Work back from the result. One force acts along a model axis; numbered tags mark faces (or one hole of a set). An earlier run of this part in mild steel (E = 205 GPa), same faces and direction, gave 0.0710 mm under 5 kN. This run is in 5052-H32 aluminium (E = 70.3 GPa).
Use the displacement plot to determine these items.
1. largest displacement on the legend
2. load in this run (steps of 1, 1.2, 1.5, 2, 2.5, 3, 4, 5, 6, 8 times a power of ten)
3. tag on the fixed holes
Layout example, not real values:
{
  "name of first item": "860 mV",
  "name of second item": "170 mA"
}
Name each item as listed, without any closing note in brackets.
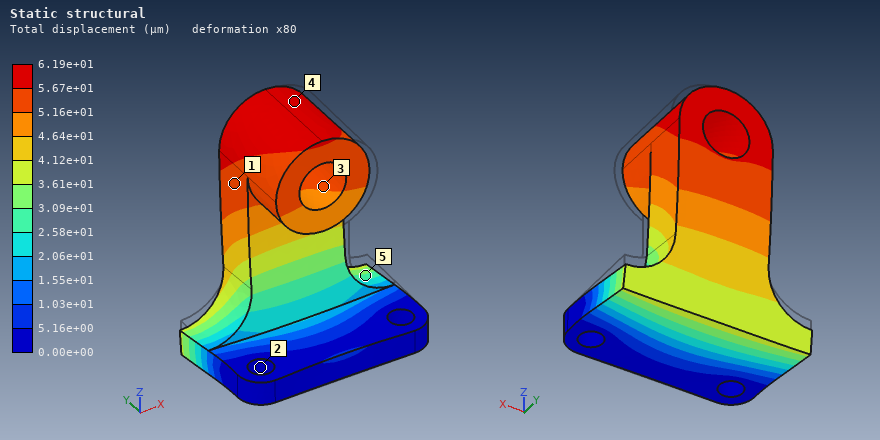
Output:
{
  "largest displacement on the legend": "6.19e+01 µm",
  "load in this run": "1.5 kN",
  "tag on the fixed holes": "2"
}
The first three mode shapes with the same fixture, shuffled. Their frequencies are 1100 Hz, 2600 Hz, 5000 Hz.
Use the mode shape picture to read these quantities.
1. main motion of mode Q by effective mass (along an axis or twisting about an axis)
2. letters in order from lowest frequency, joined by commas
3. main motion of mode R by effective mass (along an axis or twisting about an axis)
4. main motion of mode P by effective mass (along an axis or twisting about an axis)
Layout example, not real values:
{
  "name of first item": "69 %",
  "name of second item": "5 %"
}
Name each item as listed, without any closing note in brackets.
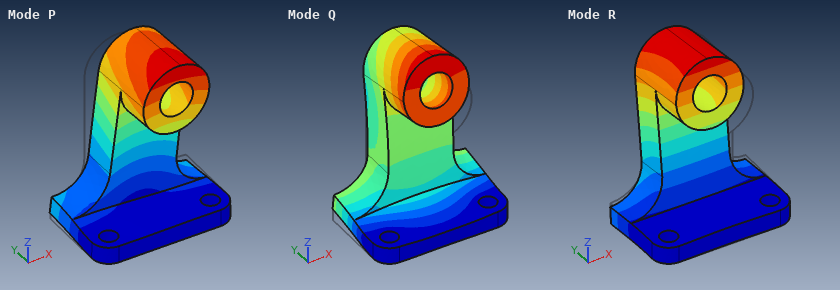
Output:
{
  "main motion of mode Q by effective mass": "along Z",
  "letters in order from lowest frequency, joined by commas": "R, P, Q",
  "main motion of mode R by effective mass": "along Y",
  "main motion of mode P by effective mass": "along X"
}
